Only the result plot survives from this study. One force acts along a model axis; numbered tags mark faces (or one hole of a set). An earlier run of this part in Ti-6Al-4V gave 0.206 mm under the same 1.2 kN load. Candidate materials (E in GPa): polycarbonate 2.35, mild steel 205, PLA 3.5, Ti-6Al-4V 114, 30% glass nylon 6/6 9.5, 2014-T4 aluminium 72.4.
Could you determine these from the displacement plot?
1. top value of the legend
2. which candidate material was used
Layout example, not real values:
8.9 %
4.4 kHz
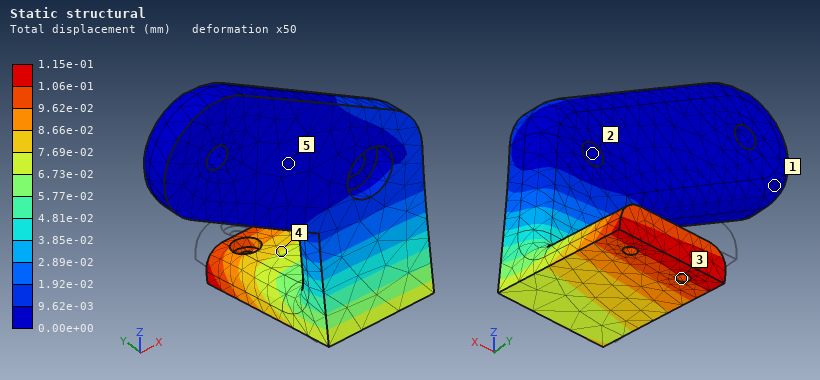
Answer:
1.15e-01 mm
mild steel
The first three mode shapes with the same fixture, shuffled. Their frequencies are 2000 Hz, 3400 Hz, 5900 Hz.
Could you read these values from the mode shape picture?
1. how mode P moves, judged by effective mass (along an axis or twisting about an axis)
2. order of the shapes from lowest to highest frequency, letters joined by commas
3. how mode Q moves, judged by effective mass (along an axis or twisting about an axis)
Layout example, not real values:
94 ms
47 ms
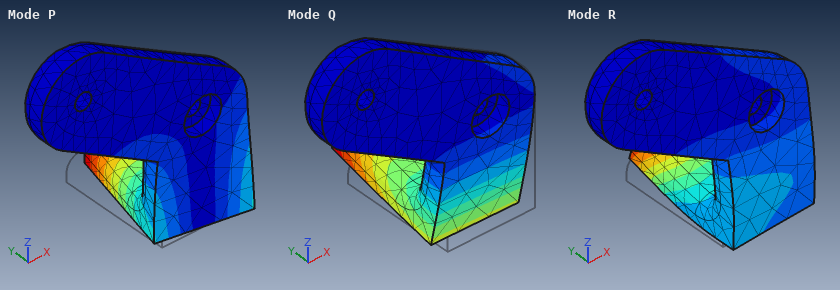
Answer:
along X
Q, P, R
along Y
